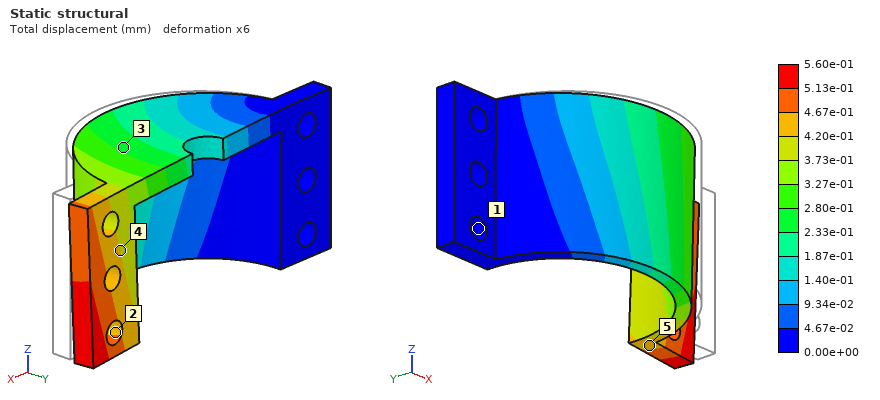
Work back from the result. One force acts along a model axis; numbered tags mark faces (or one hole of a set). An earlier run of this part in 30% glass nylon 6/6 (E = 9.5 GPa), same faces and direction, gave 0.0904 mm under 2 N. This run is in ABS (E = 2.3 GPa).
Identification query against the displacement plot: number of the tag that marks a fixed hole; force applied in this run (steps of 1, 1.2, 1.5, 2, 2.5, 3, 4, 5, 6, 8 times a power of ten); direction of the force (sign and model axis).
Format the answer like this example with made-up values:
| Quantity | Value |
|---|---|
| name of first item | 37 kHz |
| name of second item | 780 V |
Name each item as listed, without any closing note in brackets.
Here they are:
| Quantity | Value |
|---|---|
| number of the tag that marks a fixed hole | 1 |
| force applied in this run | 3 N |
| direction of the force | +Y |
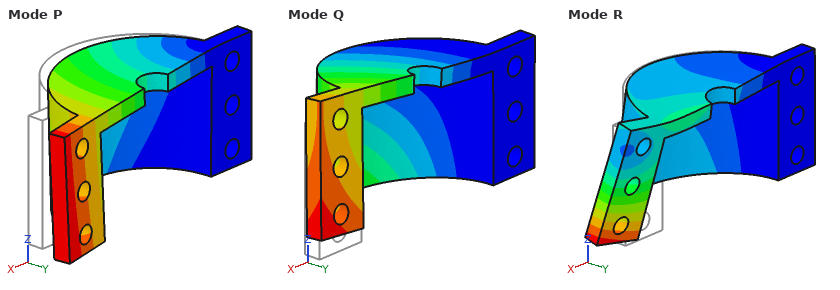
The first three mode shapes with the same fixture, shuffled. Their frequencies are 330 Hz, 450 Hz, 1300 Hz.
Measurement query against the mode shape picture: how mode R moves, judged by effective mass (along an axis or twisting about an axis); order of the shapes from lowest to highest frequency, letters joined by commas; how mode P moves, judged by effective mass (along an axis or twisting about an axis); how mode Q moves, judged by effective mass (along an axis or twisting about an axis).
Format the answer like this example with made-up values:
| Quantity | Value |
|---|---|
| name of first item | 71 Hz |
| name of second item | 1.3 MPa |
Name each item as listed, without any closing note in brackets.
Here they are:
| Quantity | Value |
|---|---|
| how mode R moves, judged by effective mass | along X |
| order of the shapes from lowest to highest frequency, letters joined by commas | P, Q, R |
| how mode P moves, judged by effective mass | along Y |
| how mode Q moves, judged by effective mass | along Z |
